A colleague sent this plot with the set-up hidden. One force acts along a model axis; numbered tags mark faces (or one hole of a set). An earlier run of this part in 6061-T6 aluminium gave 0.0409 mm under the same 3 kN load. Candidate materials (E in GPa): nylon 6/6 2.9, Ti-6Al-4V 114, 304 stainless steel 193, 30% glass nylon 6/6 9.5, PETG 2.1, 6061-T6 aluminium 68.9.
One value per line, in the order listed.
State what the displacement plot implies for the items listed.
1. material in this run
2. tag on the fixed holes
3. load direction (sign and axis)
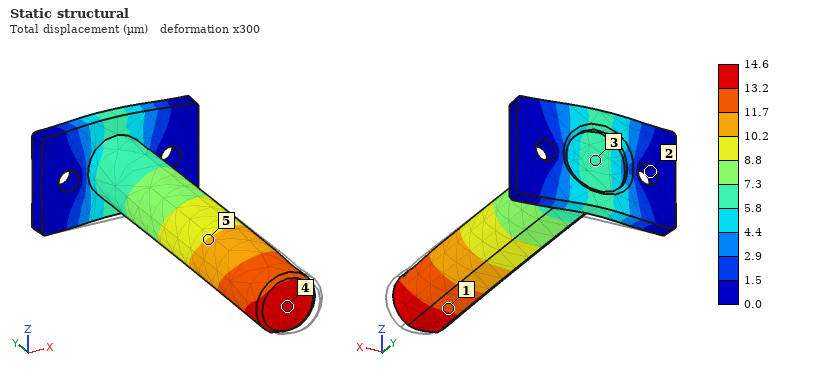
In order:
304 stainless steel
2
+Y
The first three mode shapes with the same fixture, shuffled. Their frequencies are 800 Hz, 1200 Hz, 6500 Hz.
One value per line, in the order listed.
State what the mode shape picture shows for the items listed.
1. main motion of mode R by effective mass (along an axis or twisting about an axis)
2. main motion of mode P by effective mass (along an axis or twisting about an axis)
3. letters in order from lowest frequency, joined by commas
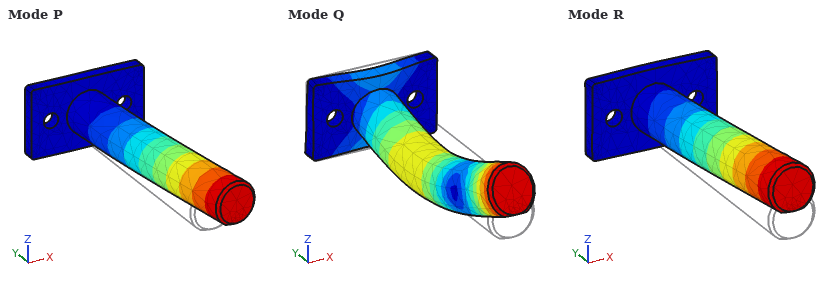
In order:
along Z
along X
R, P, Q
